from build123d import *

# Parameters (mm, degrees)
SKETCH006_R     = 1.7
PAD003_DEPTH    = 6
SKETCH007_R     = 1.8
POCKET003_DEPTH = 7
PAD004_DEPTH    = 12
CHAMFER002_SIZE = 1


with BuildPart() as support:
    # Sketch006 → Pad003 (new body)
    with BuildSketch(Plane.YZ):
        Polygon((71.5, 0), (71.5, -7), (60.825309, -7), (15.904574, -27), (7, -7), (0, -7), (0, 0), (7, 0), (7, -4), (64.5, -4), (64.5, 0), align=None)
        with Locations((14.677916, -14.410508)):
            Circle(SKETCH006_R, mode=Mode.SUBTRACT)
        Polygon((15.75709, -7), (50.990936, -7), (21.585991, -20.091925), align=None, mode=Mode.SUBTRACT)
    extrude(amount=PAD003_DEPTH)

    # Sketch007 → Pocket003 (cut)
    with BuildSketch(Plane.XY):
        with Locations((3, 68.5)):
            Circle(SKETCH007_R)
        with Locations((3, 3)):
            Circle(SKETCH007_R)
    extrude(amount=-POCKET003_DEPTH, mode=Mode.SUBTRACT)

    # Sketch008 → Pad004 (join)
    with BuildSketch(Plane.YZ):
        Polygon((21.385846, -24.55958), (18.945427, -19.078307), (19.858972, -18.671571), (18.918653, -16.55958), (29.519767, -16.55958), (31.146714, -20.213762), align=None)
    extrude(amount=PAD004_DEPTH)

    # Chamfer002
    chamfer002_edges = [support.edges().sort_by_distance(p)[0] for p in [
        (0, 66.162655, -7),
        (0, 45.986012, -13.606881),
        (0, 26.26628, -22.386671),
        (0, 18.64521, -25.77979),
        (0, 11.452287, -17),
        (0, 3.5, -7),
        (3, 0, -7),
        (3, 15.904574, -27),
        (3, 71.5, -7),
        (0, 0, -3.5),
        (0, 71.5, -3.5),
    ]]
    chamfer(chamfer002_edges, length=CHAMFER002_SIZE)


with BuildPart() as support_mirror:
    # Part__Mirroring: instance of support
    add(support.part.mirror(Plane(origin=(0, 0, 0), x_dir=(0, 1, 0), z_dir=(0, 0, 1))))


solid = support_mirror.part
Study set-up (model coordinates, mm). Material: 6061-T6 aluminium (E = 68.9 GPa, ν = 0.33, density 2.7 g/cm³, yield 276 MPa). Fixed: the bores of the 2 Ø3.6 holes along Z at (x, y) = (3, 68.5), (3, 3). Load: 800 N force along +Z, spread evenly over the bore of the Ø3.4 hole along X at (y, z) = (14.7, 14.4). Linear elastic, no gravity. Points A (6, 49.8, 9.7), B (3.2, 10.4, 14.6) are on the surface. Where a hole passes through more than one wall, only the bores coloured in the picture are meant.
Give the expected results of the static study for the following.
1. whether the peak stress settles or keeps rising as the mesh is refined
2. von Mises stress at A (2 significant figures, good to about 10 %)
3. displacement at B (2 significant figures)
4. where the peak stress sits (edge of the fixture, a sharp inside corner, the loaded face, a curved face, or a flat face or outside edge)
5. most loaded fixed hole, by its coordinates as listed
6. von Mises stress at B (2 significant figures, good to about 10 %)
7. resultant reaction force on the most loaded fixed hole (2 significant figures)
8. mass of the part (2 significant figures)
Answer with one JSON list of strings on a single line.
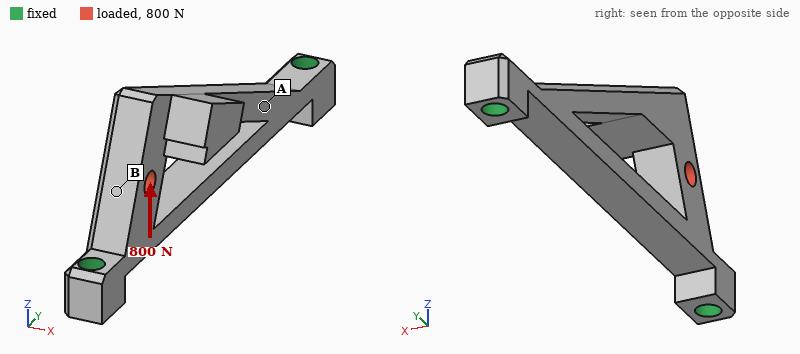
["keeps rising", "12 MPa", "17 µm", "edge of the fixture", "(3, 3)", "59 MPa", "740 N", "10 g"]
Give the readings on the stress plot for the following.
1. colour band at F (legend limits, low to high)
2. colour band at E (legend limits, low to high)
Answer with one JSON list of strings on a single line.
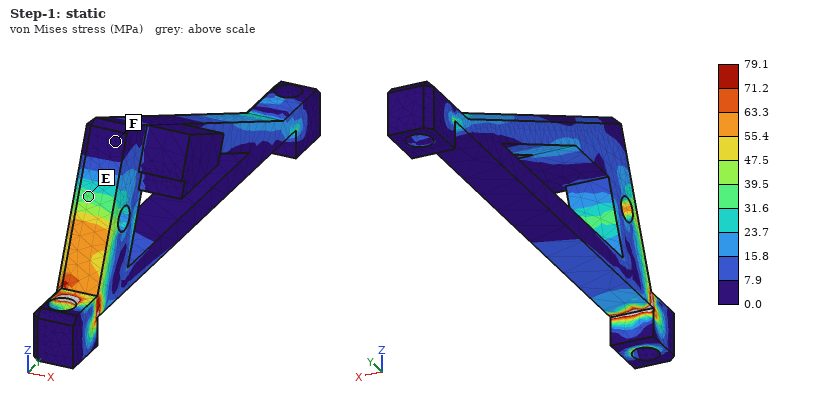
["0.0 to 7.9 MPa", "31.6 to 39.5 MPa"]
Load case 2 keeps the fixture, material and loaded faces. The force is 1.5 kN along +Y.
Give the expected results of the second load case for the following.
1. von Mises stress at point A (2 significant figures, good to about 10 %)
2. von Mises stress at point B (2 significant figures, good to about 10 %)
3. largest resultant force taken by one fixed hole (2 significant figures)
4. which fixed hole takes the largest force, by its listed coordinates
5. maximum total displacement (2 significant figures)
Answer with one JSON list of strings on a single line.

["28 MPa", "66 MPa", "920 N", "(3, 3)", "30 µm"]
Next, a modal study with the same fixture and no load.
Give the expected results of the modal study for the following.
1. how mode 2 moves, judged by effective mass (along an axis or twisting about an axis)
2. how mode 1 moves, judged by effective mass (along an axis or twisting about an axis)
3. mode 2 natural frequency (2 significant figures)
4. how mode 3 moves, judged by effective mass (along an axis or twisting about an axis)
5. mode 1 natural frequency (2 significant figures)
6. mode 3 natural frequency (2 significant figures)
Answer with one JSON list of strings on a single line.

["along Z", "along X", "6000 Hz", "along X", "3200 Hz", "7200 Hz"]
